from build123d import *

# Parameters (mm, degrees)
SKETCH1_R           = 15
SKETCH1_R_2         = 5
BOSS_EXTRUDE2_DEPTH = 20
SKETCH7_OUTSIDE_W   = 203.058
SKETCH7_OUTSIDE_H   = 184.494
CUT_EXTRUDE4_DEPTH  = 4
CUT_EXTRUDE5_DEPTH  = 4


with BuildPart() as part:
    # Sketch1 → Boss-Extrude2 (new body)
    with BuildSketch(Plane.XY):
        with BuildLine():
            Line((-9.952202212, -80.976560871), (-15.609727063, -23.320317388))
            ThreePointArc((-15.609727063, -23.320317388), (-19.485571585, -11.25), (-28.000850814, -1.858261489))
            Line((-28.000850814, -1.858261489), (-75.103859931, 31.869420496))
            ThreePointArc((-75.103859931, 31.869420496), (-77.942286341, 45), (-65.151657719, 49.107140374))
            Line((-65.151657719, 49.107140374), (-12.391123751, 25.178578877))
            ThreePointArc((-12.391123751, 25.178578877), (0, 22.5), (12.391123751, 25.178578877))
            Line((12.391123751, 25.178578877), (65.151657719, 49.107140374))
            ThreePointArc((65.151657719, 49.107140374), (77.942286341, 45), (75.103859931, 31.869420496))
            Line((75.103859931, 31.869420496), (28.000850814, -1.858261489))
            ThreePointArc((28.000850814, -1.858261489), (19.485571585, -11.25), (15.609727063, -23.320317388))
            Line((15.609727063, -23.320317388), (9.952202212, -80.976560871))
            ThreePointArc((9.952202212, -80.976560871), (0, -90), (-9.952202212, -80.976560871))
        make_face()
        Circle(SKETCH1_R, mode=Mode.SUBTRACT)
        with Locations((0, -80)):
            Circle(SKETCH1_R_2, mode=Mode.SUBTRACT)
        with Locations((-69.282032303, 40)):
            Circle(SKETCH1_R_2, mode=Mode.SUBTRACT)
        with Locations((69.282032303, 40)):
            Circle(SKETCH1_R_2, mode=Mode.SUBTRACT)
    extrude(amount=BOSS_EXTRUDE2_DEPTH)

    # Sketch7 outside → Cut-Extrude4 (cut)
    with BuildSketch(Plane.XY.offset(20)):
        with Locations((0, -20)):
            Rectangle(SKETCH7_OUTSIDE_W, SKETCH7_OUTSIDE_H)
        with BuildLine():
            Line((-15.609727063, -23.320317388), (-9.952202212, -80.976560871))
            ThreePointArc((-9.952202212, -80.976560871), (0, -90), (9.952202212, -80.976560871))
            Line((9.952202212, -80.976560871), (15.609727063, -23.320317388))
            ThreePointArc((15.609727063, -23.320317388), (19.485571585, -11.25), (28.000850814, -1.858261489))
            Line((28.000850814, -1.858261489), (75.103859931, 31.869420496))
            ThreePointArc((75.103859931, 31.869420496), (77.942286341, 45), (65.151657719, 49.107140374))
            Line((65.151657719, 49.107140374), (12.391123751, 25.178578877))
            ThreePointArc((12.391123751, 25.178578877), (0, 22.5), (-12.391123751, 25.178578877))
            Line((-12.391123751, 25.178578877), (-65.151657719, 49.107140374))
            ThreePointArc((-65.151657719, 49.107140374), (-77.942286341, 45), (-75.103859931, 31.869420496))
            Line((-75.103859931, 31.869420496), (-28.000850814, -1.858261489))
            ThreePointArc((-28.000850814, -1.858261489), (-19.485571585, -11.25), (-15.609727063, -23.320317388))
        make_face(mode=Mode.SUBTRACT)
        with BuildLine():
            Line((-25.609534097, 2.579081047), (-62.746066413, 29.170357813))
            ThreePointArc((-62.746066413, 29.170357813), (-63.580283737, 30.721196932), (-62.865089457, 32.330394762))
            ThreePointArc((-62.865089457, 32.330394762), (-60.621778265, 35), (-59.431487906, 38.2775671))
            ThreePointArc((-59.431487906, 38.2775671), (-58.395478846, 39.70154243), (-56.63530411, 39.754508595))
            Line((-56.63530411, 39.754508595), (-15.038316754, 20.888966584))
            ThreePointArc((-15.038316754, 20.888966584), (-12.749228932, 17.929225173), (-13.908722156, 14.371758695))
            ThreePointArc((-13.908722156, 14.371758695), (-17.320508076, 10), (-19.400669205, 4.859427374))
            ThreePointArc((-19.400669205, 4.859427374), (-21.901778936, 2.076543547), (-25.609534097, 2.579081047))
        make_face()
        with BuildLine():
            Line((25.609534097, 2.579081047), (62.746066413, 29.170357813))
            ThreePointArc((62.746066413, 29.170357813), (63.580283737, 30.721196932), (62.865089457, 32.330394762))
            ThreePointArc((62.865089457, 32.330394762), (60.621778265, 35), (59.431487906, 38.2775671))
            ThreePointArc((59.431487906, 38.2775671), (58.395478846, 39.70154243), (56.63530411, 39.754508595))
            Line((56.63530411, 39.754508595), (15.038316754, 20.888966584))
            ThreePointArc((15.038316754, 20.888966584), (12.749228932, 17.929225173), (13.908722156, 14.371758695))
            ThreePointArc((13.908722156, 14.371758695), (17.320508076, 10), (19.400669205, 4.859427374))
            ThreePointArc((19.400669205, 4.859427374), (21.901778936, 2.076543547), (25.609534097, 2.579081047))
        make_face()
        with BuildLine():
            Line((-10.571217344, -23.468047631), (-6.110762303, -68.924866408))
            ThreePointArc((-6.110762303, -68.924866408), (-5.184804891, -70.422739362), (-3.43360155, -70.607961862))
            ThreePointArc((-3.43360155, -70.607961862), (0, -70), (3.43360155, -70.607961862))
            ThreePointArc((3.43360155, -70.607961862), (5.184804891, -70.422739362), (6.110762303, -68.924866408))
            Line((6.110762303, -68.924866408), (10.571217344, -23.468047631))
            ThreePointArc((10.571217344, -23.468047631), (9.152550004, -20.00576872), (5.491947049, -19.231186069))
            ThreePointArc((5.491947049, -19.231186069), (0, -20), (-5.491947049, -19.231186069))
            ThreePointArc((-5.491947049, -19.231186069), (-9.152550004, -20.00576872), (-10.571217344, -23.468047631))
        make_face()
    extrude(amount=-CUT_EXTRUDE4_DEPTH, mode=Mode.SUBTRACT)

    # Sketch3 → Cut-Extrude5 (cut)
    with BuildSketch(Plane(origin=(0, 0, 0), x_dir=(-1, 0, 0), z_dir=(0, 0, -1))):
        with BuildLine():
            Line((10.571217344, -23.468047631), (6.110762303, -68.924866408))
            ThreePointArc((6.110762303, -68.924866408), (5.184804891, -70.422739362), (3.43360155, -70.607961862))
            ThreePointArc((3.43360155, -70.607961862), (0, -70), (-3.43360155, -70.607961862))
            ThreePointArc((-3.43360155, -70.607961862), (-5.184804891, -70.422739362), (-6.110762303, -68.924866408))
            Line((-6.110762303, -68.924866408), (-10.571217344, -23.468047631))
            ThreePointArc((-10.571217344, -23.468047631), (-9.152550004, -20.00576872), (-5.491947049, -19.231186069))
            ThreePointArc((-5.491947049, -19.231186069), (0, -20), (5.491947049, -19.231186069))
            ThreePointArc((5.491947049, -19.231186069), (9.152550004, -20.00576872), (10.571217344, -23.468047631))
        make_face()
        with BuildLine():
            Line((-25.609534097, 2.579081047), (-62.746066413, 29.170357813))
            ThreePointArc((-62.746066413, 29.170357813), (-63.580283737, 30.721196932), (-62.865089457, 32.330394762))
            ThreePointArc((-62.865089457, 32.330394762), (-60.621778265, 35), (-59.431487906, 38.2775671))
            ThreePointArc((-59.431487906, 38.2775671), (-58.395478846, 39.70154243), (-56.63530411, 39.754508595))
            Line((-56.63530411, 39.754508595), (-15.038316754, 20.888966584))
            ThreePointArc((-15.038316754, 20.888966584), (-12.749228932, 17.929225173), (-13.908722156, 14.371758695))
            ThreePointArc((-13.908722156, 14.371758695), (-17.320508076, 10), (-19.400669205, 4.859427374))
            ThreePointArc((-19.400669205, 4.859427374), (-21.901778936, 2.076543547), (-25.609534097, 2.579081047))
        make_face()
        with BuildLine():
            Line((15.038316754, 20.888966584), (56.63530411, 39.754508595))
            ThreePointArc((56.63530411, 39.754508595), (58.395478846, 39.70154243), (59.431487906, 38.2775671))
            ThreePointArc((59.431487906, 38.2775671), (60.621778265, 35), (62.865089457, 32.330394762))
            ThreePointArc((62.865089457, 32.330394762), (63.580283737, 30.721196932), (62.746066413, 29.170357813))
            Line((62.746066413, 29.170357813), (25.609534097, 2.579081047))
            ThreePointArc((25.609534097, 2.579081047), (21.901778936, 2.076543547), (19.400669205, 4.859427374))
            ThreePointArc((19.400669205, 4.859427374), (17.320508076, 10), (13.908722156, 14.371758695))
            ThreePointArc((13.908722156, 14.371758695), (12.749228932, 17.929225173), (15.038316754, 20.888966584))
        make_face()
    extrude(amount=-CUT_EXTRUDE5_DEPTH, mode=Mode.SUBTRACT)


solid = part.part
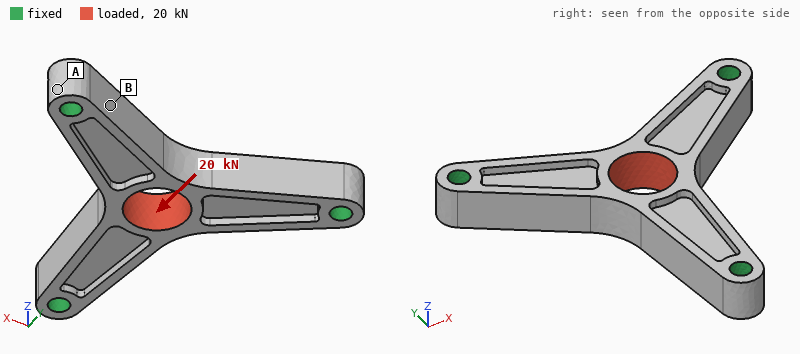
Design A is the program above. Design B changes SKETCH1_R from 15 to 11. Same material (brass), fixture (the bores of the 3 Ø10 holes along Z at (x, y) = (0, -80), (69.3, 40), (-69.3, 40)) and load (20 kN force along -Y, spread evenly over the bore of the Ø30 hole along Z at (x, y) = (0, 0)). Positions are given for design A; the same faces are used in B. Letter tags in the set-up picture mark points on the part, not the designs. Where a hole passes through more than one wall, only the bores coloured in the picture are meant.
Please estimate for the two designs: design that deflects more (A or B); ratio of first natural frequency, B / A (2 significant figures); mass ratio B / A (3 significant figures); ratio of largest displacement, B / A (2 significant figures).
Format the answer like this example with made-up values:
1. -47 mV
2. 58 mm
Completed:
1. A
2. 0.96
3. 1.07
4. 0.67
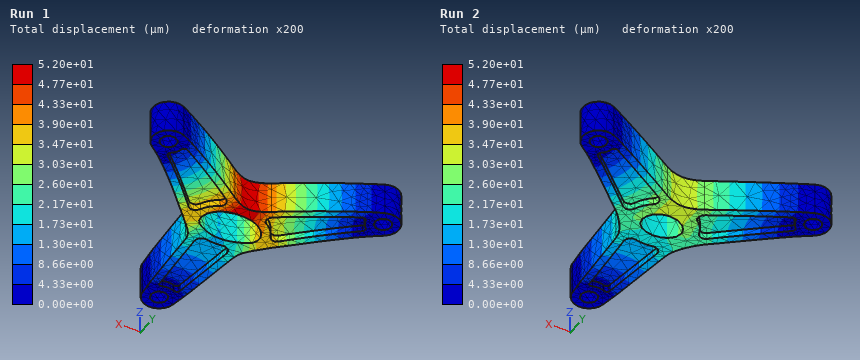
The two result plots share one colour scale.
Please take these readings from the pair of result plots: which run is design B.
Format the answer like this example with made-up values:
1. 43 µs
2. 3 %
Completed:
1. Run 2
